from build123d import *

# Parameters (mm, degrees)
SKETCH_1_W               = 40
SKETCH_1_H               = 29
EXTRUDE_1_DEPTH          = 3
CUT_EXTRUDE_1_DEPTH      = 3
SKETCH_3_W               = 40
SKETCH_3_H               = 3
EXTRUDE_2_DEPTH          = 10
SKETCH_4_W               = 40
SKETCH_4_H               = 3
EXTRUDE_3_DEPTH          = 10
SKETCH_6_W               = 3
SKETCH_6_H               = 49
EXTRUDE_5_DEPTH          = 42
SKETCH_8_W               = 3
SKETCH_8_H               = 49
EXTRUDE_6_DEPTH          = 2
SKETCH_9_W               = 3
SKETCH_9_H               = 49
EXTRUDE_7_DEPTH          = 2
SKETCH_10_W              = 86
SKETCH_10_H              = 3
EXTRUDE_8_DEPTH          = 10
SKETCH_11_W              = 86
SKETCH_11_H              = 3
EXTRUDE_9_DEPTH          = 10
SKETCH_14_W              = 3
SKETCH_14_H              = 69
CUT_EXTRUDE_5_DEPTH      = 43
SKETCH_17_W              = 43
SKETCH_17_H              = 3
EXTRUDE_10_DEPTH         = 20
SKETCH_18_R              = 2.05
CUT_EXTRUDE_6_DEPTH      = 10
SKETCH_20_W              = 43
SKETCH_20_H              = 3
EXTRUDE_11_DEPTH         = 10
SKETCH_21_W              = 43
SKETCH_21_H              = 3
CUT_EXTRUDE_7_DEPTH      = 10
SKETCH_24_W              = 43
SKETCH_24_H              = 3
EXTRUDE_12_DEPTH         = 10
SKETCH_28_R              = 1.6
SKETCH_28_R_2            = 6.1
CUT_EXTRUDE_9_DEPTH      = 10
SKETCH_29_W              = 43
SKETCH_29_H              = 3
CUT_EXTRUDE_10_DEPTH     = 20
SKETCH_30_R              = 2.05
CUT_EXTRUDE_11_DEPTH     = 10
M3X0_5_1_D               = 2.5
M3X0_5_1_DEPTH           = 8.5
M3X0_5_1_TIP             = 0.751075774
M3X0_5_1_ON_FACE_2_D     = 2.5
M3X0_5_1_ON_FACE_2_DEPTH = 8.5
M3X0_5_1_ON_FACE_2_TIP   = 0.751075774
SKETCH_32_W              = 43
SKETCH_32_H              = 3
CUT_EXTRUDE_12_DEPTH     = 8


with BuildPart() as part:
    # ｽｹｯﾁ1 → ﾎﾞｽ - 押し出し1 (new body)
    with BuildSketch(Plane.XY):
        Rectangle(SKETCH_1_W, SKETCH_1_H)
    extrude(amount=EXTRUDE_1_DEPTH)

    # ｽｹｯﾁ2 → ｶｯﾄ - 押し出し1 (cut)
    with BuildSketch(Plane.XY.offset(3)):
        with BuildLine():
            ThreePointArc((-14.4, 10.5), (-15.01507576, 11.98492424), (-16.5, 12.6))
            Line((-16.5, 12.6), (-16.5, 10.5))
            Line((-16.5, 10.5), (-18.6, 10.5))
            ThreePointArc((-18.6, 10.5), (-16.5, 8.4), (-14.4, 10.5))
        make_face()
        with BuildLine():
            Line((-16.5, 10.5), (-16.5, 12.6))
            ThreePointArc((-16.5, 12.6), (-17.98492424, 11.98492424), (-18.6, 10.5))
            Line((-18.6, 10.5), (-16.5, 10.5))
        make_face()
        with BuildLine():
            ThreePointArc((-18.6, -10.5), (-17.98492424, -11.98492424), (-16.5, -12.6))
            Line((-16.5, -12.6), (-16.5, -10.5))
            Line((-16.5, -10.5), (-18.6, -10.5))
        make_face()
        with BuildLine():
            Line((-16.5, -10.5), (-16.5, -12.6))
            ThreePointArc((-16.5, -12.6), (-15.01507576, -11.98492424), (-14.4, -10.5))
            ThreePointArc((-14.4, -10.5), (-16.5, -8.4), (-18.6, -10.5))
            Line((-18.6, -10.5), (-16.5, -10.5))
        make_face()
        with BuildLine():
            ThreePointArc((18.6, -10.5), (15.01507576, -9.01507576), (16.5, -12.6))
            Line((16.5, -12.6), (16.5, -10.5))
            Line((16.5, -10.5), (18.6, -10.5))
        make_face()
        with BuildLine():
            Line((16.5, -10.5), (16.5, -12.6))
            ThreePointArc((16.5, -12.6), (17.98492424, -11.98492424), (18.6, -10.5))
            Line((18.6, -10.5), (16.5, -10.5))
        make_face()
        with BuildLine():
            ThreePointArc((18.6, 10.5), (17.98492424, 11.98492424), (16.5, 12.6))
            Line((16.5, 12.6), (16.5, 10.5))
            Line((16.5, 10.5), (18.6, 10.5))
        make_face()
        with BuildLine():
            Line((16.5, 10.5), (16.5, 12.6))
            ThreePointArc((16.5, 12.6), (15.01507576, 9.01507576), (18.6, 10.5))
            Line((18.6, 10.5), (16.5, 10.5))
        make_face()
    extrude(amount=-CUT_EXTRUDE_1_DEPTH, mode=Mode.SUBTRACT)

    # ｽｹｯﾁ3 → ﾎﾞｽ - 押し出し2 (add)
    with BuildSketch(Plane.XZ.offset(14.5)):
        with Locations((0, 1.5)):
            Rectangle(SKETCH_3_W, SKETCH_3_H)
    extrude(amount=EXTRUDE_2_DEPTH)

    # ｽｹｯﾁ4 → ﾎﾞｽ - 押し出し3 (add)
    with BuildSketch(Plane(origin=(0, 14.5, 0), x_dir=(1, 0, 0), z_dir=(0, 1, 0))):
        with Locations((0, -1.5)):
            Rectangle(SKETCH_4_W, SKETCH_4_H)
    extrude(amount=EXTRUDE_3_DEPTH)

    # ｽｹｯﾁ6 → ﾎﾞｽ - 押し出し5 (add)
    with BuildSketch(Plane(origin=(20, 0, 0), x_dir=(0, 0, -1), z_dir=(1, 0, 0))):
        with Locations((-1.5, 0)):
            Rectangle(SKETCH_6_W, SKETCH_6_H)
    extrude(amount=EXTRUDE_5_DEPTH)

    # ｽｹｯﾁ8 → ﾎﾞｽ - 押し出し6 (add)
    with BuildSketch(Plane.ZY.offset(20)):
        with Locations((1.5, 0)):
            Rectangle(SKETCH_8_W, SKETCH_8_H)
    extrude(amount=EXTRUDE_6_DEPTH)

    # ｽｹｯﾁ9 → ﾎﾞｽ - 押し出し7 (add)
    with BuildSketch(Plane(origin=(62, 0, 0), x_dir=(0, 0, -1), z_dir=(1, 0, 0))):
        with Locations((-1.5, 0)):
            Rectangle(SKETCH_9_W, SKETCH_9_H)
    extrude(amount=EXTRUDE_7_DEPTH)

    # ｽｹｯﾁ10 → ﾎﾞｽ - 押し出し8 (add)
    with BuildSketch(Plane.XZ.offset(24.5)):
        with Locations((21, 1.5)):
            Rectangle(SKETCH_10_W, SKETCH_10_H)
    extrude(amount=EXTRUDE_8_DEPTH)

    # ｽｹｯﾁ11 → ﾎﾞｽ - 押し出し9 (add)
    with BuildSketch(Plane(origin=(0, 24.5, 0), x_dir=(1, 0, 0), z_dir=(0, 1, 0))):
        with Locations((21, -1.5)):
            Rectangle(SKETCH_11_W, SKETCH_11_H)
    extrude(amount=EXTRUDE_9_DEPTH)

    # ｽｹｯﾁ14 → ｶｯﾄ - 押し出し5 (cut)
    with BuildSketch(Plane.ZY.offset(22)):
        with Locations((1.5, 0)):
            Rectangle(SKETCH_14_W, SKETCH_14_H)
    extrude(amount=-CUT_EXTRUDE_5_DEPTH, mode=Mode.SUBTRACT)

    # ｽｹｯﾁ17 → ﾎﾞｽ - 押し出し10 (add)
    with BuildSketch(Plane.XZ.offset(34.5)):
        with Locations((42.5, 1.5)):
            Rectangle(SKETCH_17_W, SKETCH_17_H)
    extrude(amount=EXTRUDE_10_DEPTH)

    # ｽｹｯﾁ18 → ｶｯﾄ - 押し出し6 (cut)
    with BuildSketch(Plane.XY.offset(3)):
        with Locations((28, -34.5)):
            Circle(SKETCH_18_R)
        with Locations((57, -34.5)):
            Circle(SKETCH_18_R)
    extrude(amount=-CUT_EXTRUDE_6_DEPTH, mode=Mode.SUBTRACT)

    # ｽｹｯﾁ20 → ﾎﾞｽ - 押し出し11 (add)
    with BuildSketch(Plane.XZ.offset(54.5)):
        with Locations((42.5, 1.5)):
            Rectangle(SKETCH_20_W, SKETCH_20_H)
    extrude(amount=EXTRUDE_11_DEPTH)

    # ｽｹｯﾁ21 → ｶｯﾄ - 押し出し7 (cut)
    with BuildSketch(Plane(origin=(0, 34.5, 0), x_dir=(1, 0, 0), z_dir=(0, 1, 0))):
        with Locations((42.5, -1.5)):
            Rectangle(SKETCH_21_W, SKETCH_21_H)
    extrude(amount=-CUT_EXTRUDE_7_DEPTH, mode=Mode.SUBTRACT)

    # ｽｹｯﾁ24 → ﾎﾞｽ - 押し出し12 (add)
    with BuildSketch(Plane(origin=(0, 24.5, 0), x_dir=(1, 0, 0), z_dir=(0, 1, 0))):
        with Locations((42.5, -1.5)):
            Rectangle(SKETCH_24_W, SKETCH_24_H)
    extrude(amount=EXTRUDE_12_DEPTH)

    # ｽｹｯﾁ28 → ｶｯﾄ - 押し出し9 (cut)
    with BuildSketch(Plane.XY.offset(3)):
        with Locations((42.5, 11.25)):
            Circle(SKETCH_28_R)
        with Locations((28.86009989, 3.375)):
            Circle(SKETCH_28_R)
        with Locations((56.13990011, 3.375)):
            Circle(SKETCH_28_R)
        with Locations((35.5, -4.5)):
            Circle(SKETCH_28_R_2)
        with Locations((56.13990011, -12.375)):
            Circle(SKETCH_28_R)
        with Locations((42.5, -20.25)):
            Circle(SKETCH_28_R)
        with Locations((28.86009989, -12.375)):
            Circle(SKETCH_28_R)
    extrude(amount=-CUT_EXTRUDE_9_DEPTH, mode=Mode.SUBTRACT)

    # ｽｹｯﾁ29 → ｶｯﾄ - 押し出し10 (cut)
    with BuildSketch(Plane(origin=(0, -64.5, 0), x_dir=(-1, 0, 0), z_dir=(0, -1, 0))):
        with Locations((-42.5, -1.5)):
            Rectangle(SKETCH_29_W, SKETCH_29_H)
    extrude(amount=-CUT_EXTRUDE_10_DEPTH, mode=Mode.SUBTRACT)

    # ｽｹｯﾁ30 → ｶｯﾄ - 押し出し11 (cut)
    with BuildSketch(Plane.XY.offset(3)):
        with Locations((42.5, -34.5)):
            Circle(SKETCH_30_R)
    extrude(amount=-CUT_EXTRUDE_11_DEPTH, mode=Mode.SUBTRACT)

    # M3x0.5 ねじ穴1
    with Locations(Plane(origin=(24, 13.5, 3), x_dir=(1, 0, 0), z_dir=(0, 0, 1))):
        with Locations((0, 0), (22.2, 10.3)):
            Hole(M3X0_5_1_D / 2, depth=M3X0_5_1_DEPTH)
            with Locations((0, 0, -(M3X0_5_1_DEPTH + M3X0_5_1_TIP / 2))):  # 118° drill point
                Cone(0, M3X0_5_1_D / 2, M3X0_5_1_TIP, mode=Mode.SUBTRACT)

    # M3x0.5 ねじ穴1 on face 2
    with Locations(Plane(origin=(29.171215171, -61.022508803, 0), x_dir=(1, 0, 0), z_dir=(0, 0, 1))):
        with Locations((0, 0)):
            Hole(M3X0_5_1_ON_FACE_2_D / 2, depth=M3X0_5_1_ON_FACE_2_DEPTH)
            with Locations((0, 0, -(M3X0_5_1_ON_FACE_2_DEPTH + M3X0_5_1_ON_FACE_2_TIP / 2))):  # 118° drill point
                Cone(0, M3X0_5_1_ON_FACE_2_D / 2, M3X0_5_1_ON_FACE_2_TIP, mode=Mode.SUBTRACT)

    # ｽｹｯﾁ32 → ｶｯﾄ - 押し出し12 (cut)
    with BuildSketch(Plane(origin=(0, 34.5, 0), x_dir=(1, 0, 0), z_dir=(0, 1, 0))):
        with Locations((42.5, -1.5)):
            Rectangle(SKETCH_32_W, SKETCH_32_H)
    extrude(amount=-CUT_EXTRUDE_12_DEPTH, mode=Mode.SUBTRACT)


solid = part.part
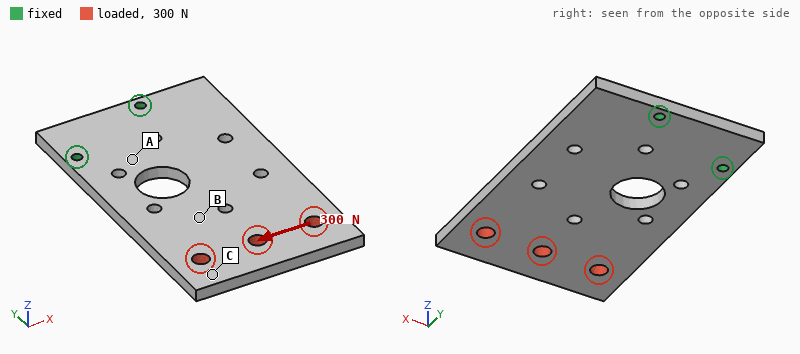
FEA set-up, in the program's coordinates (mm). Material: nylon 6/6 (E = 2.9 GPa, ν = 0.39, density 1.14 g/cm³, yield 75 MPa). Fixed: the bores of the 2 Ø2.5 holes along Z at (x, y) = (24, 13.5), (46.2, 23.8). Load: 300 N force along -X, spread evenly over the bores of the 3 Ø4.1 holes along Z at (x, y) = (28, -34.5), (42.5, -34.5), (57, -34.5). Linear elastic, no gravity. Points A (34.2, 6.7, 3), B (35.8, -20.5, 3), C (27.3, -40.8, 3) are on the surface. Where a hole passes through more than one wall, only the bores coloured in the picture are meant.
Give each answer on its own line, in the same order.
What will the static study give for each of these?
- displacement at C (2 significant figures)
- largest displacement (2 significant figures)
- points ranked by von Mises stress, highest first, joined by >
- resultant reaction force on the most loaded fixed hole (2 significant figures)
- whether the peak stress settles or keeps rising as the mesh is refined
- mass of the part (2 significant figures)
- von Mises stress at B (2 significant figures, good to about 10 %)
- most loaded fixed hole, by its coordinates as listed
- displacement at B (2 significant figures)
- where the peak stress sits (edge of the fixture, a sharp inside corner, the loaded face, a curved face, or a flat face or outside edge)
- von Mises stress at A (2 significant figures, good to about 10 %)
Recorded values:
0.86 mm
0.98 mm
A > B > C
700 N
keeps rising
9.7 g
7.9 MPa
(24, 13.5)
0.54 mm
edge of the fixture
17 MPa
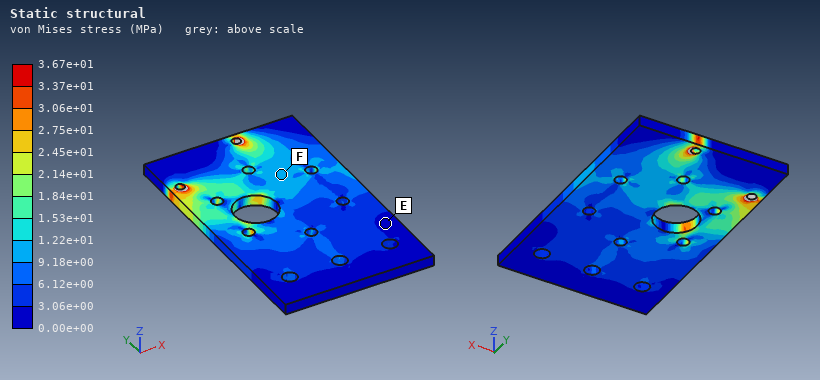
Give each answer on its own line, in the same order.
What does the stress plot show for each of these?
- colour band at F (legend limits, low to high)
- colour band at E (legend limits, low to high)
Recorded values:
9.18e+00 to 1.22e+01 MPa
0.00e+00 to 3.06e+00 MPa
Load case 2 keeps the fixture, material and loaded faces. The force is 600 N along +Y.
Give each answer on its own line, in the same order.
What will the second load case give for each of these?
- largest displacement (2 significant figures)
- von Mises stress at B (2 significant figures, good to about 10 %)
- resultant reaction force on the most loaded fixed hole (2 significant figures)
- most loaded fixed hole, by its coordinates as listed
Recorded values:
0.26 mm
3.3 MPa
450 N
(46.2, 23.8)
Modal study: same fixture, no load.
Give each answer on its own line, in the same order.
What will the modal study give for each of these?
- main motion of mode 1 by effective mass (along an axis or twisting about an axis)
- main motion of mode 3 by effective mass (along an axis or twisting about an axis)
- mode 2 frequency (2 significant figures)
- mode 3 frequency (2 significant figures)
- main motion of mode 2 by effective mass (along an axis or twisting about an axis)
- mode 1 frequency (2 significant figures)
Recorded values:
along Z
along Z
540 Hz
1100 Hz
twisting about Y
170 Hz
